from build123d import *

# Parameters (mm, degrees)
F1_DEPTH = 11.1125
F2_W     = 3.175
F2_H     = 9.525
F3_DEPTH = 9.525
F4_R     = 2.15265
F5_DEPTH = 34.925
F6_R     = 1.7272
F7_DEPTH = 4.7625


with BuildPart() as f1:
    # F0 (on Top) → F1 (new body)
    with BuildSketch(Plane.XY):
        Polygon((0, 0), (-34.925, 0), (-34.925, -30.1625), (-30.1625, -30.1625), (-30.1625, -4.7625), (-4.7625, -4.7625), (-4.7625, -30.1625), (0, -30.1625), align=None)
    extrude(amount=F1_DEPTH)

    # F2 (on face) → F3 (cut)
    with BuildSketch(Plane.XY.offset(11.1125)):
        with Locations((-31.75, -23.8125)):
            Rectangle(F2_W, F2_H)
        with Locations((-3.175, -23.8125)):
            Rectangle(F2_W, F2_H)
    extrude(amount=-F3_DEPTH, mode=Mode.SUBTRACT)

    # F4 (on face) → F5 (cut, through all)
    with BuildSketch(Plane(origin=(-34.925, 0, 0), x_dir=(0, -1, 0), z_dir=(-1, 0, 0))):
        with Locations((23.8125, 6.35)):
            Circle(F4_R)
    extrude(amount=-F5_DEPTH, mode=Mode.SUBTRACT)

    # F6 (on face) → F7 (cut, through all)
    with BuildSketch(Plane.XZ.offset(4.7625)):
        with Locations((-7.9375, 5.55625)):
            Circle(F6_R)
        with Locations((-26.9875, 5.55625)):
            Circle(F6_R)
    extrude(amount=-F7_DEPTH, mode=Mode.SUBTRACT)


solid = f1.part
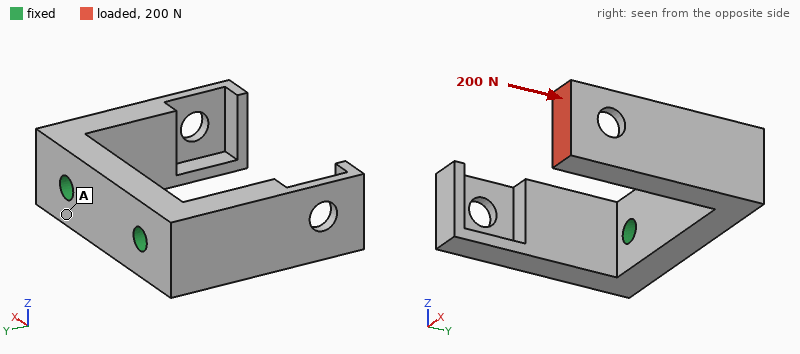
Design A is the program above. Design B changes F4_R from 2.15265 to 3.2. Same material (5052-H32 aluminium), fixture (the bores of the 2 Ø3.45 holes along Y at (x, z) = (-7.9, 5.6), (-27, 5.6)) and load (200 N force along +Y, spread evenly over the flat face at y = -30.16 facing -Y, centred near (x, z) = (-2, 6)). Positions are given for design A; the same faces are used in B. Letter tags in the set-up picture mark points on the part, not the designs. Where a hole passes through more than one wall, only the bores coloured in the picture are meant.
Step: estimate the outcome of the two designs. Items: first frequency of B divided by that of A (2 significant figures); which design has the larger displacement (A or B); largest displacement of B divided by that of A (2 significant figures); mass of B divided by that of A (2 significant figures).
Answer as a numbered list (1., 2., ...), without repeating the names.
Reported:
1. 1.0
2. B
3. 1.2
4. 0.99
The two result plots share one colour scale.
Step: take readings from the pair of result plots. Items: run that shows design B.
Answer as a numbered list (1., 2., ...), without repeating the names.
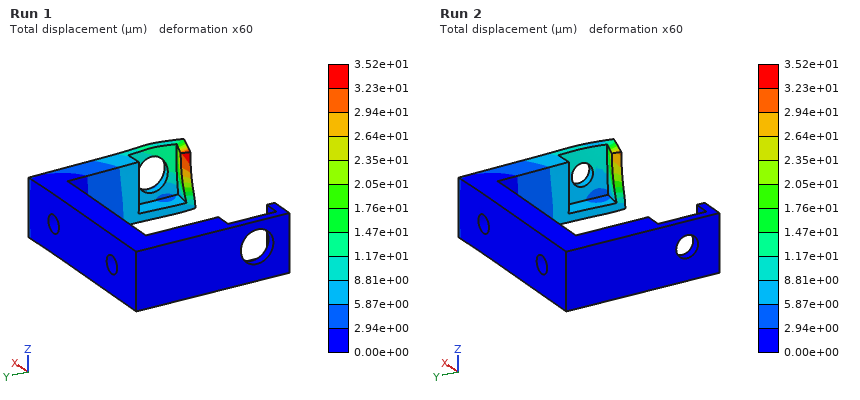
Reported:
1. Run 1
